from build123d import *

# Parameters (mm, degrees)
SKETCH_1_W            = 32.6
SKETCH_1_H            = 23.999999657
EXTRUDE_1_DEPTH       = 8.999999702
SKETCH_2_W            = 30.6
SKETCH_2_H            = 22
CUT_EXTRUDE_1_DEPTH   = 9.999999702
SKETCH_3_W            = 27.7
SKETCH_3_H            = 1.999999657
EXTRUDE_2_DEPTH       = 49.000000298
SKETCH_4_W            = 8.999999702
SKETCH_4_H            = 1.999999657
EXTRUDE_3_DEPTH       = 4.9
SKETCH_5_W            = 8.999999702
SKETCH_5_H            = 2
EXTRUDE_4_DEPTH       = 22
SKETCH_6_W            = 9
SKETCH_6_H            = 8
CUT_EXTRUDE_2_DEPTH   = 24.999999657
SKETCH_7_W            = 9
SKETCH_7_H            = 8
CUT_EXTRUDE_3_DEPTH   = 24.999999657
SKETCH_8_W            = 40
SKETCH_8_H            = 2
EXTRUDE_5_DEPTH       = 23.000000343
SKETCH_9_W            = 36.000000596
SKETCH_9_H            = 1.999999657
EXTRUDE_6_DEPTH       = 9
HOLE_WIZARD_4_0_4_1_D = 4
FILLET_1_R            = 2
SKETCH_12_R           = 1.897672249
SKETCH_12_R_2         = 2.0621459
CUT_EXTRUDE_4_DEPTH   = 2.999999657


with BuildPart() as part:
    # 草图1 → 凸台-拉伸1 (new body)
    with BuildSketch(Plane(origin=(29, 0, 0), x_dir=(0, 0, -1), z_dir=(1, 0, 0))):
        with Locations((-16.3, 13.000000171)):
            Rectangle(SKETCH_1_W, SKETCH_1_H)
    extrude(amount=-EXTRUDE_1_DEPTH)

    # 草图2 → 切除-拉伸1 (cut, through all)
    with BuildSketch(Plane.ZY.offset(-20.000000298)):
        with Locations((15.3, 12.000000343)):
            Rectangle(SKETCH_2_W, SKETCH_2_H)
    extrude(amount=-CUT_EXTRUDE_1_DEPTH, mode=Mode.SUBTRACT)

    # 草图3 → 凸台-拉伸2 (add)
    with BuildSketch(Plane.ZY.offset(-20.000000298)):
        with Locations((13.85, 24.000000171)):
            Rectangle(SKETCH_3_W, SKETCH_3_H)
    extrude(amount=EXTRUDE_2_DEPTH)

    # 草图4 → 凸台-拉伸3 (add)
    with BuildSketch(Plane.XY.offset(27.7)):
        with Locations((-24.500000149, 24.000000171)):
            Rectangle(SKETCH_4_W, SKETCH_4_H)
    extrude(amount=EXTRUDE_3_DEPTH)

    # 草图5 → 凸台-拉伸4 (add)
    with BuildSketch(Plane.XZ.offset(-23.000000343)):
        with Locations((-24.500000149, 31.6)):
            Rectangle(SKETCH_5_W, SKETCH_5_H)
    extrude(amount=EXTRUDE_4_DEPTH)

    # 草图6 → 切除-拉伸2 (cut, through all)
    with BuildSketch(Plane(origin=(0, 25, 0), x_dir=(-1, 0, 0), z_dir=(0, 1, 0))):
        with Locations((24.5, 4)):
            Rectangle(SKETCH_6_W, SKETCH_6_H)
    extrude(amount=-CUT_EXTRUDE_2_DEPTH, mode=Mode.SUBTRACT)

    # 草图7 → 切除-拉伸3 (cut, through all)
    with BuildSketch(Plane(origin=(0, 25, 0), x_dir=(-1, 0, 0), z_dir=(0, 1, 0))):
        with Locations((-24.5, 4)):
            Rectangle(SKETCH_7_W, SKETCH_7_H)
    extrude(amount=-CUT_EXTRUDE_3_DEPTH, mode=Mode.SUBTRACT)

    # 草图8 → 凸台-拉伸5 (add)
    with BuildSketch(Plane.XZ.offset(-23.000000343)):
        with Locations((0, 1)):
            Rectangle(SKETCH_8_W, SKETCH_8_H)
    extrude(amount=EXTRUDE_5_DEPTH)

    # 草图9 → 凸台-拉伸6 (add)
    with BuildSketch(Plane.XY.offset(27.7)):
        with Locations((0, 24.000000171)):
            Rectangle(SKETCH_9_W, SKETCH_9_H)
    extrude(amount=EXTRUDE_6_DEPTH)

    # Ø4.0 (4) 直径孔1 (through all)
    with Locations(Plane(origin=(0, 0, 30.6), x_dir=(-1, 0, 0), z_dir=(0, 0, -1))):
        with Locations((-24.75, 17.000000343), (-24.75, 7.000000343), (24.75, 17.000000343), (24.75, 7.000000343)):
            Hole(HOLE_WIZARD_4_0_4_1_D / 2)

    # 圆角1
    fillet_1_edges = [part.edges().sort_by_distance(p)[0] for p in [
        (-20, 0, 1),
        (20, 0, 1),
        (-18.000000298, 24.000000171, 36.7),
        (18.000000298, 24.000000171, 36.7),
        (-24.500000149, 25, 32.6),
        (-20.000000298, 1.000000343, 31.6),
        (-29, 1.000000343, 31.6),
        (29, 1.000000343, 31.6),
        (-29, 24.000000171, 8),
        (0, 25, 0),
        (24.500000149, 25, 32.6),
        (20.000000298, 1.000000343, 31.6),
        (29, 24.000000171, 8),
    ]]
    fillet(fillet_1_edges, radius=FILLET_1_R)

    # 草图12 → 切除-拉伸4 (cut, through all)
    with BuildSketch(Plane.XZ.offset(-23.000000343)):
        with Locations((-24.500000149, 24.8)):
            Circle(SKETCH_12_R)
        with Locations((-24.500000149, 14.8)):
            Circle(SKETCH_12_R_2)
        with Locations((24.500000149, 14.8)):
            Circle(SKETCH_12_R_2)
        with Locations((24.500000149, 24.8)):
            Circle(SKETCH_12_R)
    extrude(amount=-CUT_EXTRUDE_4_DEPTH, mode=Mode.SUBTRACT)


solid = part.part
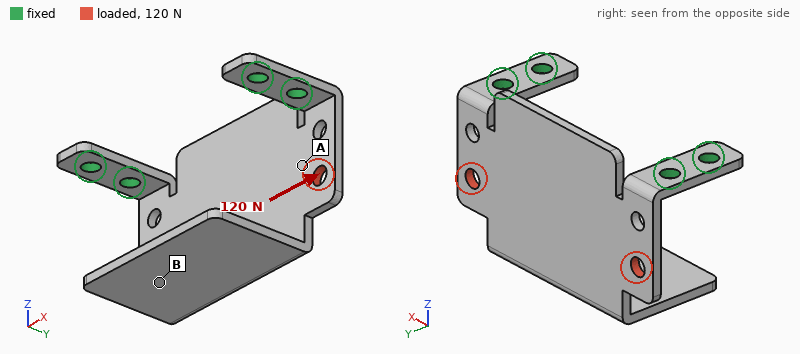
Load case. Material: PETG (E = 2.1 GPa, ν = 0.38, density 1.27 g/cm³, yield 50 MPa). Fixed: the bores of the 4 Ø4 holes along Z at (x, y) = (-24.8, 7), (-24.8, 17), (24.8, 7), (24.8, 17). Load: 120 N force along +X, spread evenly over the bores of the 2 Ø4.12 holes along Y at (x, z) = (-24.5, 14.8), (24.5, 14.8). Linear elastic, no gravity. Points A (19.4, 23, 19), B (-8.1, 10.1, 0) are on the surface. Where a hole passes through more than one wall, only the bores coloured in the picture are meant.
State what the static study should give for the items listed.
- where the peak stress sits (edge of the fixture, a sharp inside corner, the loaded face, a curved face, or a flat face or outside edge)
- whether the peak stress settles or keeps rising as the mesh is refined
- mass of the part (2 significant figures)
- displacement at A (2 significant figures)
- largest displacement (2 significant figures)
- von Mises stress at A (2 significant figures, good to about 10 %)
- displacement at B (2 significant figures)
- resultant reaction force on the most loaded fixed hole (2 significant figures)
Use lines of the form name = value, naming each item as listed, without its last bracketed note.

where the peak stress sits = edge of the fixture
whether the peak stress settles or keeps rising as the mesh is refined = keeps rising
mass of the part = 7.8 g
displacement at A = 0.34 mm
largest displacement = 0.79 mm
von Mises stress at A = 5.0 MPa
displacement at B = 0.58 mm
resultant reaction force on the most loaded fixed hole = 80 N
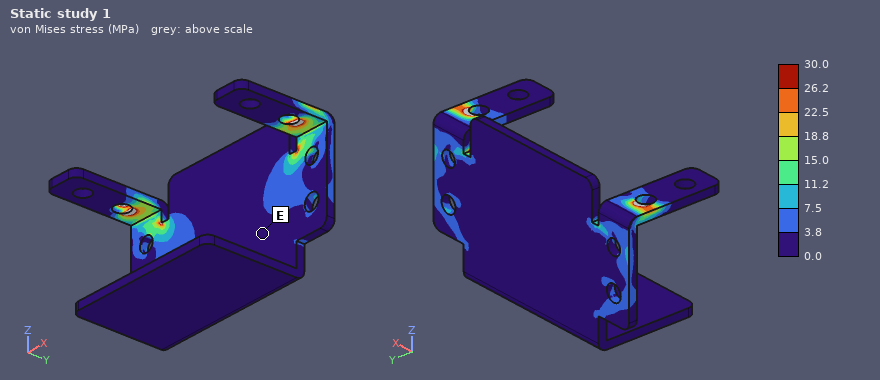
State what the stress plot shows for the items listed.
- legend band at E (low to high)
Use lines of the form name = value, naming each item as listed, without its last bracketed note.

legend band at E = 0.0 to 3.8 MPa
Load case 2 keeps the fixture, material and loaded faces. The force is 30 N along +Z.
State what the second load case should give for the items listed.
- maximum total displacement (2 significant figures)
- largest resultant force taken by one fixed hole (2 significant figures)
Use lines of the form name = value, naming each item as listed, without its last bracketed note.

maximum total displacement = 0.67 mm
largest resultant force taken by one fixed hole = 15 N
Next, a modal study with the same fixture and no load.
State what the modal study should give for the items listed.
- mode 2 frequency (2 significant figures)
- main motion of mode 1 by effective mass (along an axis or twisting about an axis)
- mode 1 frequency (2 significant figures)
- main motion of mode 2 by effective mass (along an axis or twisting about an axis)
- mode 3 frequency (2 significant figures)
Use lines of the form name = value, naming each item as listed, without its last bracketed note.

mode 2 frequency = 340 Hz
main motion of mode 1 by effective mass = along Y
mode 1 frequency = 110 Hz
main motion of mode 2 by effective mass = along X
mode 3 frequency = 450 Hz
